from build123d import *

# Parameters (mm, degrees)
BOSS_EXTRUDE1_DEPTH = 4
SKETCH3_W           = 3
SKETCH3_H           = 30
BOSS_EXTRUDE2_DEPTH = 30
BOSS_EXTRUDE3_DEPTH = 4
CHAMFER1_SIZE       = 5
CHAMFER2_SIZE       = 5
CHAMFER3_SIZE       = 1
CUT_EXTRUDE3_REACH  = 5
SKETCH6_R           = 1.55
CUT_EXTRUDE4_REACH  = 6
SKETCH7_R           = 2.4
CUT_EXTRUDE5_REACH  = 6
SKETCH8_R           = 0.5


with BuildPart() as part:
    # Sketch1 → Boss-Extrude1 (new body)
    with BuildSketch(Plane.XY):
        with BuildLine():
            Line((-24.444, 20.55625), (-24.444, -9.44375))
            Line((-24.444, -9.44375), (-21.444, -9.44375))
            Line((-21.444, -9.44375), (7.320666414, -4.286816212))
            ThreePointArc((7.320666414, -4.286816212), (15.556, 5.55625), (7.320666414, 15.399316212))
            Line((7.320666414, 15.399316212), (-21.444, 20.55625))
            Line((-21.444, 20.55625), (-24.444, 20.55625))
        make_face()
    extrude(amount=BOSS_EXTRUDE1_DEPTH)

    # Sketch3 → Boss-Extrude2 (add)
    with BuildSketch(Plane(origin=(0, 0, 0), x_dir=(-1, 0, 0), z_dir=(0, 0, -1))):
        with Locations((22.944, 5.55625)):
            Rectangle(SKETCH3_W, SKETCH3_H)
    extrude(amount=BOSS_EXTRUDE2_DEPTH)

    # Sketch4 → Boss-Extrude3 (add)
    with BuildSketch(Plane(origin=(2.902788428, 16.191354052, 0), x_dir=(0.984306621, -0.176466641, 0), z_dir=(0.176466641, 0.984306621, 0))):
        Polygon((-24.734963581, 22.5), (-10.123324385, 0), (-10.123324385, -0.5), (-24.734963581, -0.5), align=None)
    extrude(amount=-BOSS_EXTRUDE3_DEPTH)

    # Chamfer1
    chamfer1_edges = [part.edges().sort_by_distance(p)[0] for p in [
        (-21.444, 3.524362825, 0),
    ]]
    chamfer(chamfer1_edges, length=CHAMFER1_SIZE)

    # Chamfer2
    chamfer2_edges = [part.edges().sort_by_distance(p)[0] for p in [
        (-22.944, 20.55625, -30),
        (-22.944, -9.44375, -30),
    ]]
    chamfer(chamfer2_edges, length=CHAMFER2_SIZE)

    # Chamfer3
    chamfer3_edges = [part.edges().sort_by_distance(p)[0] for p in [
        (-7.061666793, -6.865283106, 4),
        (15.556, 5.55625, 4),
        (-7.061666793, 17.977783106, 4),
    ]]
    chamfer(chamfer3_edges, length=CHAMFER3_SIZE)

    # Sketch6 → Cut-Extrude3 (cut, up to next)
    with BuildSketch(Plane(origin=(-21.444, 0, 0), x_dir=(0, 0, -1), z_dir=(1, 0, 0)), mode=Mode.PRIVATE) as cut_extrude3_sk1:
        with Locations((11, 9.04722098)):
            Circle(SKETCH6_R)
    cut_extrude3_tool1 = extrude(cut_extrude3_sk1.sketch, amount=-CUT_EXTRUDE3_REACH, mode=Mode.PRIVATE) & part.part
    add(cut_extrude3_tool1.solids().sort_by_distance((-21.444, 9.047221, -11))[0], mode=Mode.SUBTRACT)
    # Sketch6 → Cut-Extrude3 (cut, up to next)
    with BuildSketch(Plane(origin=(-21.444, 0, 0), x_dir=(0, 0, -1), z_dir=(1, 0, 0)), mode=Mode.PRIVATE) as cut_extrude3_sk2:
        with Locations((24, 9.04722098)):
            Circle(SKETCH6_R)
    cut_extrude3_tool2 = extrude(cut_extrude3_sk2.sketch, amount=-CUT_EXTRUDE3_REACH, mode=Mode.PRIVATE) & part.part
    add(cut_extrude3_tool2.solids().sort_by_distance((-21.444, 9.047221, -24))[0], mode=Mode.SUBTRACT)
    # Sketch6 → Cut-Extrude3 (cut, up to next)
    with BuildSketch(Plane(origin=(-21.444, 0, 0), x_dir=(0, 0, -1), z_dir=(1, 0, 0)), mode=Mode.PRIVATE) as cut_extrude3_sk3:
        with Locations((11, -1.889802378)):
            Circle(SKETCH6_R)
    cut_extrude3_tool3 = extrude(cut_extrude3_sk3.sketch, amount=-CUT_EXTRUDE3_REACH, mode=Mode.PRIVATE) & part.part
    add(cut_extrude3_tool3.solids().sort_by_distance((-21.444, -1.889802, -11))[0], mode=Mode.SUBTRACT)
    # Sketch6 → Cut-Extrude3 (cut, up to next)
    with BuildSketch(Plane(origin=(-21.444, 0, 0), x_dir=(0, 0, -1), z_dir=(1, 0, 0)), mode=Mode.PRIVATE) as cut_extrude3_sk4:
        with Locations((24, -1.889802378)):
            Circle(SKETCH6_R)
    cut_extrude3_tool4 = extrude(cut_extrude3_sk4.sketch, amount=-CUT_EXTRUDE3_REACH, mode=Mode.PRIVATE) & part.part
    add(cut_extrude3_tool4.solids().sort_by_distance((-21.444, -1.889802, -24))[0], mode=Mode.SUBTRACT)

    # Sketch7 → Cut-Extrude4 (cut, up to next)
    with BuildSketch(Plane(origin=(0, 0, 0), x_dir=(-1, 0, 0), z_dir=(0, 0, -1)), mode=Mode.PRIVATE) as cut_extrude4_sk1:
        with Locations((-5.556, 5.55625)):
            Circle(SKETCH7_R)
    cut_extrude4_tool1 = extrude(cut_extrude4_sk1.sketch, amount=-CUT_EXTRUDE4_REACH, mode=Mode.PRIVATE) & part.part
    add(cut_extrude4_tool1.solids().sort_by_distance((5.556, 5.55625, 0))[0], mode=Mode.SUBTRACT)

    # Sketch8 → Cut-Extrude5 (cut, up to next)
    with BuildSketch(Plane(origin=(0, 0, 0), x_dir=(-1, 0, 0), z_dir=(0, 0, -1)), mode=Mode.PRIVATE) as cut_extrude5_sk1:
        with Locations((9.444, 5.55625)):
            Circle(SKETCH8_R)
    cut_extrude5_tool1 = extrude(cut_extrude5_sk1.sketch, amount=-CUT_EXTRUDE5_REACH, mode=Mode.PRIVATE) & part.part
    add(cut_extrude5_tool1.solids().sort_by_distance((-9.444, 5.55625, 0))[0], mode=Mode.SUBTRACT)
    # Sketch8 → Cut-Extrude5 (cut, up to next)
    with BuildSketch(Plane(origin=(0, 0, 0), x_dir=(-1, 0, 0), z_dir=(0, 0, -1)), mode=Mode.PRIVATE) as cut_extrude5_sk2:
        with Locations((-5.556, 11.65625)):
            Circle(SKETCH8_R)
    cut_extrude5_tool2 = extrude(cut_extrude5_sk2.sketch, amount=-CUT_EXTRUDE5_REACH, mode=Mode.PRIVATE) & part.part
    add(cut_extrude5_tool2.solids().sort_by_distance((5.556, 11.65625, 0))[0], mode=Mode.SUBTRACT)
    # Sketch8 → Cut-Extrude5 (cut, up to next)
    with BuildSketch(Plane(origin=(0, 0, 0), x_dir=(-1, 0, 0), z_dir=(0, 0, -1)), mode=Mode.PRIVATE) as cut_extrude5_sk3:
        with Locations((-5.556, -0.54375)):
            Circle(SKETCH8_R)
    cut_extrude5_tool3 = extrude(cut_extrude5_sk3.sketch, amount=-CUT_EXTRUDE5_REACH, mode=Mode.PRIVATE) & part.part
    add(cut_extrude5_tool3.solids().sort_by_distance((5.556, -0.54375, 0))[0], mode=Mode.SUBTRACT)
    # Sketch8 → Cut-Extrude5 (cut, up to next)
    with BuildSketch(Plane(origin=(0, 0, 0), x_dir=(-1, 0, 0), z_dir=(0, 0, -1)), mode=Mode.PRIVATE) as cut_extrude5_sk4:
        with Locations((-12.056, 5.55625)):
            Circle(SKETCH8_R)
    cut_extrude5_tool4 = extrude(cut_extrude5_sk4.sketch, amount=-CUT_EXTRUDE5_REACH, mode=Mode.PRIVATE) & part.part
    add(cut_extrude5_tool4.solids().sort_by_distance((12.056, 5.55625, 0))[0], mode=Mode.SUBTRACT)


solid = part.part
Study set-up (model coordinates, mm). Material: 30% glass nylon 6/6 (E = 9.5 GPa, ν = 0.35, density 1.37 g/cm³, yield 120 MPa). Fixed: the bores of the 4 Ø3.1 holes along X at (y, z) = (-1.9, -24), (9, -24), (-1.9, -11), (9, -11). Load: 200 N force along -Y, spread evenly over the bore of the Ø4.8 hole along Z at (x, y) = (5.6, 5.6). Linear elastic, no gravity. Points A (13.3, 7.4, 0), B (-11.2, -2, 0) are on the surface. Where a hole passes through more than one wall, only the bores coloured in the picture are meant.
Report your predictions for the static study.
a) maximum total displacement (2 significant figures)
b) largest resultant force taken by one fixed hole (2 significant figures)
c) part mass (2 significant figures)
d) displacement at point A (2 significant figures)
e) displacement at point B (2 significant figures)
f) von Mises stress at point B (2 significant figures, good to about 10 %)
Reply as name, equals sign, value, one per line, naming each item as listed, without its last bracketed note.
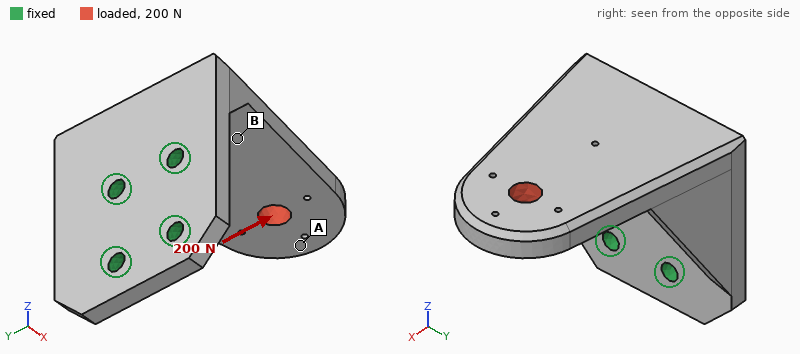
maximum total displacement = 0.66 mm
largest resultant force taken by one fixed hole = 410 N
part mass = 9.7 g
displacement at point A = 0.62 mm
displacement at point B = 0.21 mm
von Mises stress at point B = 16 MPa
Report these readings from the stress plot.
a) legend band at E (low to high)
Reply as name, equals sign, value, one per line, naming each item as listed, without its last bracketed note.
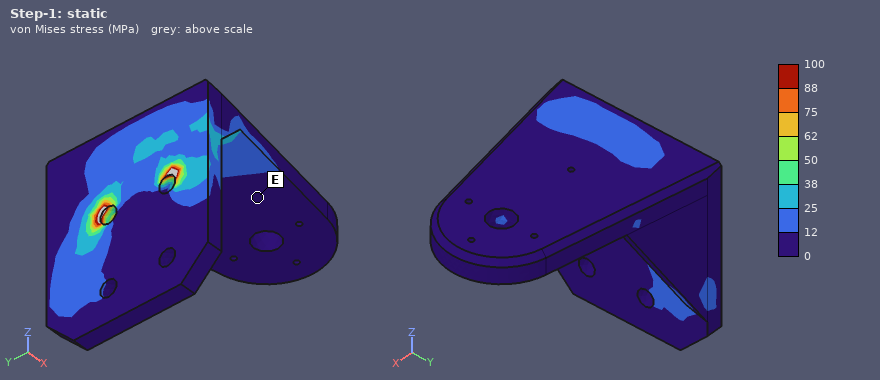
legend band at E = 0 to 12 MPa
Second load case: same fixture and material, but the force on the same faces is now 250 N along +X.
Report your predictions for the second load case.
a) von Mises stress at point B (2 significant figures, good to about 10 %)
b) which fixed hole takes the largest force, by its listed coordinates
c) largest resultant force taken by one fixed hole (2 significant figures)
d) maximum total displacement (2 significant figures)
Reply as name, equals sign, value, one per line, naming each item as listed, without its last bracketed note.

von Mises stress at point B = 5.2 MPa
which fixed hole takes the largest force, by its listed coordinates = (9, -11)
largest resultant force taken by one fixed hole = 280 N
maximum total displacement = 0.53 mm
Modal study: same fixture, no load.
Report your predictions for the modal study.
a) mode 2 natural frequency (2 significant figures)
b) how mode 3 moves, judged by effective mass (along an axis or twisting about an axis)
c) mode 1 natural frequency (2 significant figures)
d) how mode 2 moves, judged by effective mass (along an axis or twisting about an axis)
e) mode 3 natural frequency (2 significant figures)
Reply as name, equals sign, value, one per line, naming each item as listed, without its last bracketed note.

mode 2 natural frequency = 2100 Hz
how mode 3 moves, judged by effective mass = along X
mode 1 natural frequency = 1300 Hz
how mode 2 moves, judged by effective mass = along Y
mode 3 natural frequency = 3800 Hz
